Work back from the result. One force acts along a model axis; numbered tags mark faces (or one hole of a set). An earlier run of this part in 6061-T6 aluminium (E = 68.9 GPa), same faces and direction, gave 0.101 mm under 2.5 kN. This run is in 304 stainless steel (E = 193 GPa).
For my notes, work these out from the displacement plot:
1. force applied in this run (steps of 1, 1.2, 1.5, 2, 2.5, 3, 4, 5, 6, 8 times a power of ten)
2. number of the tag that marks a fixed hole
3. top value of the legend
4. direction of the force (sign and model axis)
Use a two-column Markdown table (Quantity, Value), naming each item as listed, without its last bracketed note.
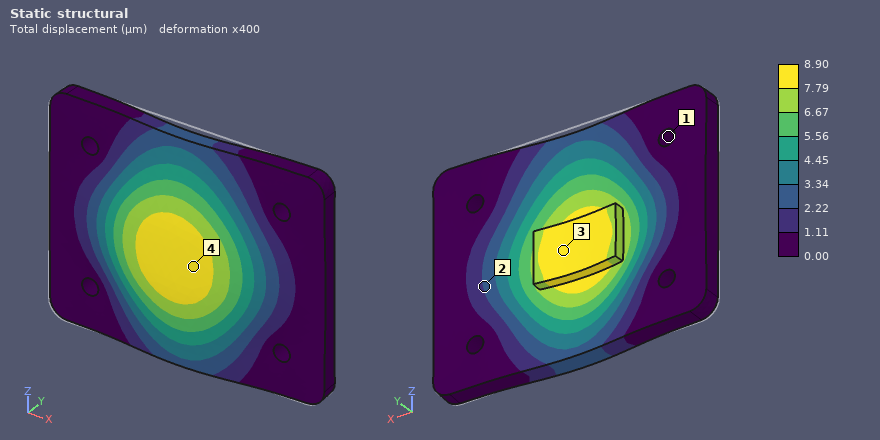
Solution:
| Quantity | Value |
|---|---|
| force applied in this run | 600 N |
| number of the tag that marks a fixed hole | 1 |
| top value of the legend | 8.90 µm |
| direction of the force | -Y |
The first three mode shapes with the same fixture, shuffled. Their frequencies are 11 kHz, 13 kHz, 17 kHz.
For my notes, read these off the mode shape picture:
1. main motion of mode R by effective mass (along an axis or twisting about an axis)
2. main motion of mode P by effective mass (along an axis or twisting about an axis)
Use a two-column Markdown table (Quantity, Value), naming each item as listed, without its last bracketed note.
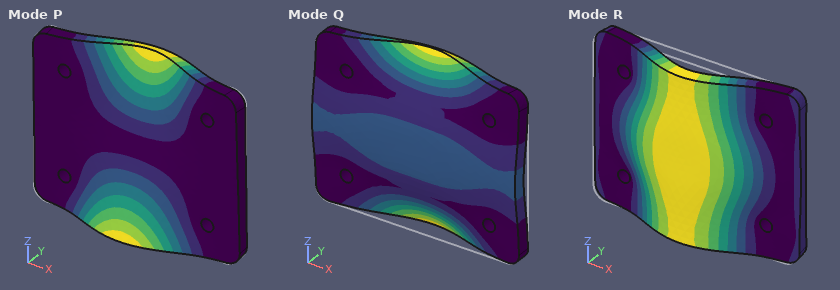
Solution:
| Quantity | Value |
|---|---|
| main motion of mode R by effective mass | along Y |
| main motion of mode P by effective mass | twisting about X |
